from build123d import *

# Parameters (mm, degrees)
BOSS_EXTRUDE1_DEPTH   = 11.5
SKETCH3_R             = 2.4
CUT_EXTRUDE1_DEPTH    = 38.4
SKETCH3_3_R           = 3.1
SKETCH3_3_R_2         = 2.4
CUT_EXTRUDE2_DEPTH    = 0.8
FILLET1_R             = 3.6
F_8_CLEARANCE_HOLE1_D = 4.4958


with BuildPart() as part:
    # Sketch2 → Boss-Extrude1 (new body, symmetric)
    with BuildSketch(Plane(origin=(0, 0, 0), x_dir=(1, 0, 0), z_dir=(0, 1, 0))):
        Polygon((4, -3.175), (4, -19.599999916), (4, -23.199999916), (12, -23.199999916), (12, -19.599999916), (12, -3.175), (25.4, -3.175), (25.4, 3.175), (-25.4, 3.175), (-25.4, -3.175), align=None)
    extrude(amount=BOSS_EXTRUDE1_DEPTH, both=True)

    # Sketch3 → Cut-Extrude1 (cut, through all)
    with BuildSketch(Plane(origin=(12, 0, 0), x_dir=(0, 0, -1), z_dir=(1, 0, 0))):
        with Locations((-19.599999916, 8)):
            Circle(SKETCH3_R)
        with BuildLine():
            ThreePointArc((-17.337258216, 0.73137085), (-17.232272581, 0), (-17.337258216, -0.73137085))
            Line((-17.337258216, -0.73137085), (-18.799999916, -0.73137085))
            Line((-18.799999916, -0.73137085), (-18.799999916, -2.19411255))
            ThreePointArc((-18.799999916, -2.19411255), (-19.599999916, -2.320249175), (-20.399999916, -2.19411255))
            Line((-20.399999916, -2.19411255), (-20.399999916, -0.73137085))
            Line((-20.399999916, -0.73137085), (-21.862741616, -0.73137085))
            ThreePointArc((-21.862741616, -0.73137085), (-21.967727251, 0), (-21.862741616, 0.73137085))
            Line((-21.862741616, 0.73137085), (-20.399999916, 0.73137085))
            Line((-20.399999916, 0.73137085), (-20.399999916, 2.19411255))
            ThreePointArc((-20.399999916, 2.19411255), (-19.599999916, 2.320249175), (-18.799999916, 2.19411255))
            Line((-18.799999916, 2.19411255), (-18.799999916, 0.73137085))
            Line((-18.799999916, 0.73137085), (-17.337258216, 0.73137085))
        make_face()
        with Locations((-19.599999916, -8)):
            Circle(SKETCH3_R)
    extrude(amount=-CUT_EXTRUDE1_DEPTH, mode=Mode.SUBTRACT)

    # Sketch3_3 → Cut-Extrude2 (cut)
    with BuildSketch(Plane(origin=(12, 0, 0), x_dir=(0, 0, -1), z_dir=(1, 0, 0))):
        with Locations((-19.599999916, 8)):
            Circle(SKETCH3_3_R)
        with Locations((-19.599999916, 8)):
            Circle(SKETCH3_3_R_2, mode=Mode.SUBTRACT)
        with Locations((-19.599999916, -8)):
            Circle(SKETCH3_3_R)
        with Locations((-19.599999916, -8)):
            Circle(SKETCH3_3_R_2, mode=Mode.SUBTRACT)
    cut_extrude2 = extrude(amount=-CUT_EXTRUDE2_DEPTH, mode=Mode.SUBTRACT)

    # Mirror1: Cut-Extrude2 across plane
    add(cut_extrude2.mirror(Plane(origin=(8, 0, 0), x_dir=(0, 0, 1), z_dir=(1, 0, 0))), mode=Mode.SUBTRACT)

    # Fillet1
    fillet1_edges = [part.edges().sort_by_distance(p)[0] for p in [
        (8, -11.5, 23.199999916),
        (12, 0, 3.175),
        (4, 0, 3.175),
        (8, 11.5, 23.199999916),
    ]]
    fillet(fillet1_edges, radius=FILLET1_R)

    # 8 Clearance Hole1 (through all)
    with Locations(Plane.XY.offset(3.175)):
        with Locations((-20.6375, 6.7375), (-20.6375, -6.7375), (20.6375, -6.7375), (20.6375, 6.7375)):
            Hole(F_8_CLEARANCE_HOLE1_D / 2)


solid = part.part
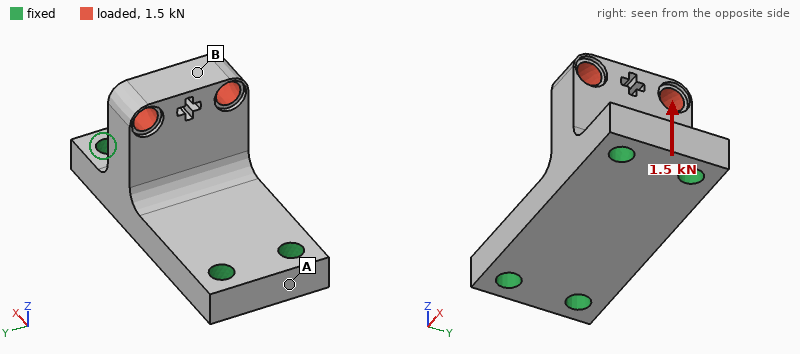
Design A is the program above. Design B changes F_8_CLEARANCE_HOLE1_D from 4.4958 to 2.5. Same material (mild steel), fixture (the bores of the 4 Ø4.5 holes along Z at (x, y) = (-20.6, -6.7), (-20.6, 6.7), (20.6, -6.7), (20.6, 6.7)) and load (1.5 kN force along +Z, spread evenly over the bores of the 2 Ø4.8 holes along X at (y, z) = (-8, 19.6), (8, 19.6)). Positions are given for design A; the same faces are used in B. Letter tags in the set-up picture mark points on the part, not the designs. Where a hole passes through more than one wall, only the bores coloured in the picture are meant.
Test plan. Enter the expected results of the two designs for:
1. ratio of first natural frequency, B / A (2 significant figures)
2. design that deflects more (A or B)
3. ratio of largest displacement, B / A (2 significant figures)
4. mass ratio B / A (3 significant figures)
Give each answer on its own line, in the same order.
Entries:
0.93
B
1.2
1.03
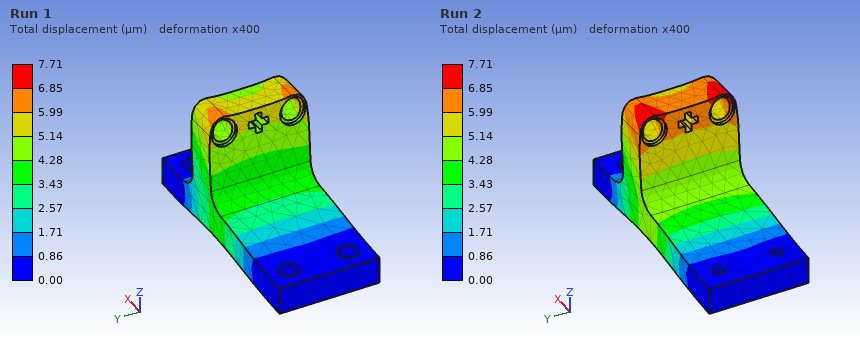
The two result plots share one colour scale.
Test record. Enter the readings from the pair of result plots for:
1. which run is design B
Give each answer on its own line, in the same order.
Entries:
Run 2
